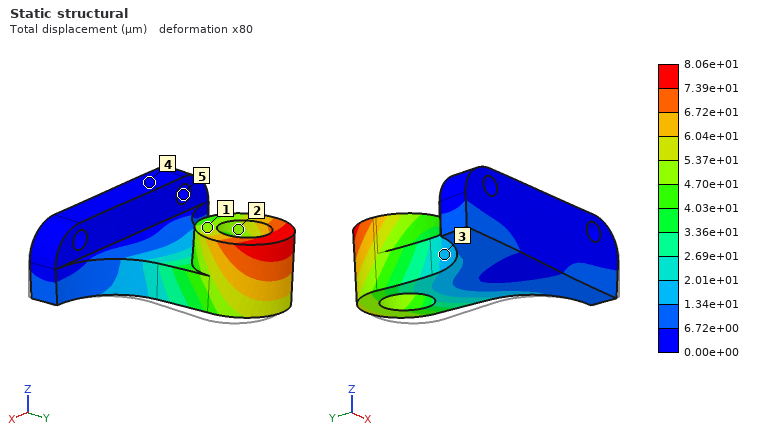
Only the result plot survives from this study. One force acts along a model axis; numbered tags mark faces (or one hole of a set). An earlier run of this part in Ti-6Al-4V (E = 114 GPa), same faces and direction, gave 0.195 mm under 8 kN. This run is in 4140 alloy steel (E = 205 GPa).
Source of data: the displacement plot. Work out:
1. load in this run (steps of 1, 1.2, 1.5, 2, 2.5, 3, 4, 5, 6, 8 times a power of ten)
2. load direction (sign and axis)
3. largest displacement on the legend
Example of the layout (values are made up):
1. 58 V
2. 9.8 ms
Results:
1. 6 kN
2. -X
3. 8.06e+01 µm
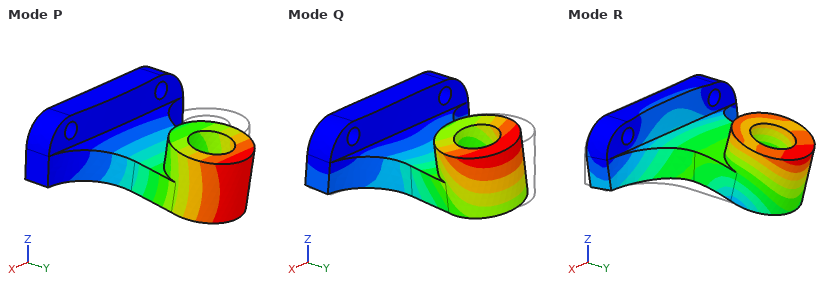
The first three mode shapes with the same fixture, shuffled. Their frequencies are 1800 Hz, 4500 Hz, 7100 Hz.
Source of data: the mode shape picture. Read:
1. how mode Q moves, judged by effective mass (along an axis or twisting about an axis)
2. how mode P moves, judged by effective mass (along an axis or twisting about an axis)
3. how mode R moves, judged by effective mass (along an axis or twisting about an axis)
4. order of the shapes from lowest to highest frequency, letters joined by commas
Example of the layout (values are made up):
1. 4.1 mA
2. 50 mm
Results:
1. along X
2. along Z
3. along Y
4. P, Q, R
